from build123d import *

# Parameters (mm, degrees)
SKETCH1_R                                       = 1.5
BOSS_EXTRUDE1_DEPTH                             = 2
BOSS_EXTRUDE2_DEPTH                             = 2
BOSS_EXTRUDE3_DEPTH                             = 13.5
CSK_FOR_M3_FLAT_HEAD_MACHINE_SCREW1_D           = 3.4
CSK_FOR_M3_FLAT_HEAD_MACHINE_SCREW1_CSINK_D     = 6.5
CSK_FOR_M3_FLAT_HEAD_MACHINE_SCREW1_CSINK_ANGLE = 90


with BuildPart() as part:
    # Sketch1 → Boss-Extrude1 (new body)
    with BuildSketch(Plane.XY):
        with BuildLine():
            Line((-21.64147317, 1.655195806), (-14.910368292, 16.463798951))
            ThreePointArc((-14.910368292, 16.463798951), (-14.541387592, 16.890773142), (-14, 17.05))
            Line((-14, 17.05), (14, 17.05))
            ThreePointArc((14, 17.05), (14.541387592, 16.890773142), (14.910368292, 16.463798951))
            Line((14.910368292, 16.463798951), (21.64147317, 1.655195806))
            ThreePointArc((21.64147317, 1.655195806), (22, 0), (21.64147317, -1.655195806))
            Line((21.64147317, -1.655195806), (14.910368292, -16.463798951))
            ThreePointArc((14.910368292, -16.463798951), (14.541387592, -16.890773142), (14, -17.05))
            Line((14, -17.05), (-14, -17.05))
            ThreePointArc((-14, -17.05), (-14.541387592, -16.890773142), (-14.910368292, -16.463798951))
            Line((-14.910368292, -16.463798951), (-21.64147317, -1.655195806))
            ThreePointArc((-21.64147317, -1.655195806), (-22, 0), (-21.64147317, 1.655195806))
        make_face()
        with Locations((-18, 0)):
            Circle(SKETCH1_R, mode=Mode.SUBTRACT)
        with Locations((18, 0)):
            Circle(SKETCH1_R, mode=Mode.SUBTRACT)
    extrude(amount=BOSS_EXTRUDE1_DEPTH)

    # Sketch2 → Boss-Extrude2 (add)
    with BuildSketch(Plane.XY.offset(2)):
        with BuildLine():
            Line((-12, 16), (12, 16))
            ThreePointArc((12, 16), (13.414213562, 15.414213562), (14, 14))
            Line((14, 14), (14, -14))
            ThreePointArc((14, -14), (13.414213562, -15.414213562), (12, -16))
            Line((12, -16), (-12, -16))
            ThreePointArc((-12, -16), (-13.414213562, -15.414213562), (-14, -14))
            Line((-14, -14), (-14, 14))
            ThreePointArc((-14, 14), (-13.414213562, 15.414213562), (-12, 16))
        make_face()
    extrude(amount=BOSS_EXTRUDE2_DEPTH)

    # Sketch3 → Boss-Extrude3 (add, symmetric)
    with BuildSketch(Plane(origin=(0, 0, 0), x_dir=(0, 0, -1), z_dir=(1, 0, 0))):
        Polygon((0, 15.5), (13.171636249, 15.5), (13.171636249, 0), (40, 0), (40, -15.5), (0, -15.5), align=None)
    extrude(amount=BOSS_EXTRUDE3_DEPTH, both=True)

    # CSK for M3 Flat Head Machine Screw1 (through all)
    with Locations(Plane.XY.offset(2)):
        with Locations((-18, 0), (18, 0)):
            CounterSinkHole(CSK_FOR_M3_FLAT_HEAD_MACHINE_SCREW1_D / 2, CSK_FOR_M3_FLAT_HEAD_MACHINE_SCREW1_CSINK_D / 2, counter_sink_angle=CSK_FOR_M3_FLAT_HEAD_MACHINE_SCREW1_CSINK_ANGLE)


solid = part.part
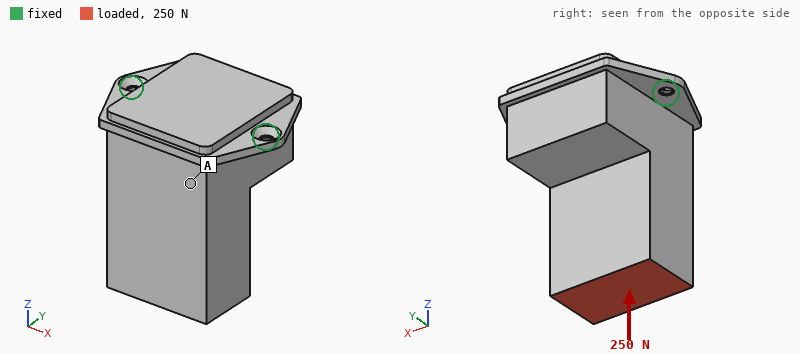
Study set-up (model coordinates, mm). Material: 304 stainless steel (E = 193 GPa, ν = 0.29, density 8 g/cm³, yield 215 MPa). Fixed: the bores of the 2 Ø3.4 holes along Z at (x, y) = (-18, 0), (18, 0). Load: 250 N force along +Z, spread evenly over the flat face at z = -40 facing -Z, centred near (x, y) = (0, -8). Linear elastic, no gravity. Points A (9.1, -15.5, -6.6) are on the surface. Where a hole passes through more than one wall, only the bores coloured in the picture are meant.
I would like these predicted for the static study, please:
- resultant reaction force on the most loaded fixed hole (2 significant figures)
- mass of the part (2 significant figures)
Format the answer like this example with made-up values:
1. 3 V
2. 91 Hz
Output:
1. 150 N
2. 210 g
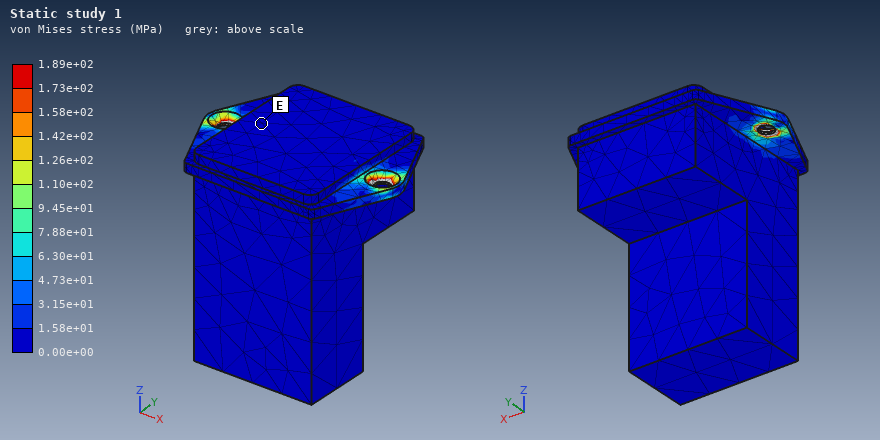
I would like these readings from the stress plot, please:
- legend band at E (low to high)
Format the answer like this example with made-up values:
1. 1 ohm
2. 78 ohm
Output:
1. 0.00e+00 to 1.58e+01 MPa
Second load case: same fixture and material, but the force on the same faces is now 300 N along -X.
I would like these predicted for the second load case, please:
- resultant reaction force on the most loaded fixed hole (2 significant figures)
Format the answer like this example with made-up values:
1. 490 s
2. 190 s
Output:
1. 400 N
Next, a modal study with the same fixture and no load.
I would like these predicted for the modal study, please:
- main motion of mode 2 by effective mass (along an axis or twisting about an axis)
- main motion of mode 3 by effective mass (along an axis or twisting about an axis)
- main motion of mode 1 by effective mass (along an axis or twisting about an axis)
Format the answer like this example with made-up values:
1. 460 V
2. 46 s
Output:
1. along X
2. along Z
3. along Y
